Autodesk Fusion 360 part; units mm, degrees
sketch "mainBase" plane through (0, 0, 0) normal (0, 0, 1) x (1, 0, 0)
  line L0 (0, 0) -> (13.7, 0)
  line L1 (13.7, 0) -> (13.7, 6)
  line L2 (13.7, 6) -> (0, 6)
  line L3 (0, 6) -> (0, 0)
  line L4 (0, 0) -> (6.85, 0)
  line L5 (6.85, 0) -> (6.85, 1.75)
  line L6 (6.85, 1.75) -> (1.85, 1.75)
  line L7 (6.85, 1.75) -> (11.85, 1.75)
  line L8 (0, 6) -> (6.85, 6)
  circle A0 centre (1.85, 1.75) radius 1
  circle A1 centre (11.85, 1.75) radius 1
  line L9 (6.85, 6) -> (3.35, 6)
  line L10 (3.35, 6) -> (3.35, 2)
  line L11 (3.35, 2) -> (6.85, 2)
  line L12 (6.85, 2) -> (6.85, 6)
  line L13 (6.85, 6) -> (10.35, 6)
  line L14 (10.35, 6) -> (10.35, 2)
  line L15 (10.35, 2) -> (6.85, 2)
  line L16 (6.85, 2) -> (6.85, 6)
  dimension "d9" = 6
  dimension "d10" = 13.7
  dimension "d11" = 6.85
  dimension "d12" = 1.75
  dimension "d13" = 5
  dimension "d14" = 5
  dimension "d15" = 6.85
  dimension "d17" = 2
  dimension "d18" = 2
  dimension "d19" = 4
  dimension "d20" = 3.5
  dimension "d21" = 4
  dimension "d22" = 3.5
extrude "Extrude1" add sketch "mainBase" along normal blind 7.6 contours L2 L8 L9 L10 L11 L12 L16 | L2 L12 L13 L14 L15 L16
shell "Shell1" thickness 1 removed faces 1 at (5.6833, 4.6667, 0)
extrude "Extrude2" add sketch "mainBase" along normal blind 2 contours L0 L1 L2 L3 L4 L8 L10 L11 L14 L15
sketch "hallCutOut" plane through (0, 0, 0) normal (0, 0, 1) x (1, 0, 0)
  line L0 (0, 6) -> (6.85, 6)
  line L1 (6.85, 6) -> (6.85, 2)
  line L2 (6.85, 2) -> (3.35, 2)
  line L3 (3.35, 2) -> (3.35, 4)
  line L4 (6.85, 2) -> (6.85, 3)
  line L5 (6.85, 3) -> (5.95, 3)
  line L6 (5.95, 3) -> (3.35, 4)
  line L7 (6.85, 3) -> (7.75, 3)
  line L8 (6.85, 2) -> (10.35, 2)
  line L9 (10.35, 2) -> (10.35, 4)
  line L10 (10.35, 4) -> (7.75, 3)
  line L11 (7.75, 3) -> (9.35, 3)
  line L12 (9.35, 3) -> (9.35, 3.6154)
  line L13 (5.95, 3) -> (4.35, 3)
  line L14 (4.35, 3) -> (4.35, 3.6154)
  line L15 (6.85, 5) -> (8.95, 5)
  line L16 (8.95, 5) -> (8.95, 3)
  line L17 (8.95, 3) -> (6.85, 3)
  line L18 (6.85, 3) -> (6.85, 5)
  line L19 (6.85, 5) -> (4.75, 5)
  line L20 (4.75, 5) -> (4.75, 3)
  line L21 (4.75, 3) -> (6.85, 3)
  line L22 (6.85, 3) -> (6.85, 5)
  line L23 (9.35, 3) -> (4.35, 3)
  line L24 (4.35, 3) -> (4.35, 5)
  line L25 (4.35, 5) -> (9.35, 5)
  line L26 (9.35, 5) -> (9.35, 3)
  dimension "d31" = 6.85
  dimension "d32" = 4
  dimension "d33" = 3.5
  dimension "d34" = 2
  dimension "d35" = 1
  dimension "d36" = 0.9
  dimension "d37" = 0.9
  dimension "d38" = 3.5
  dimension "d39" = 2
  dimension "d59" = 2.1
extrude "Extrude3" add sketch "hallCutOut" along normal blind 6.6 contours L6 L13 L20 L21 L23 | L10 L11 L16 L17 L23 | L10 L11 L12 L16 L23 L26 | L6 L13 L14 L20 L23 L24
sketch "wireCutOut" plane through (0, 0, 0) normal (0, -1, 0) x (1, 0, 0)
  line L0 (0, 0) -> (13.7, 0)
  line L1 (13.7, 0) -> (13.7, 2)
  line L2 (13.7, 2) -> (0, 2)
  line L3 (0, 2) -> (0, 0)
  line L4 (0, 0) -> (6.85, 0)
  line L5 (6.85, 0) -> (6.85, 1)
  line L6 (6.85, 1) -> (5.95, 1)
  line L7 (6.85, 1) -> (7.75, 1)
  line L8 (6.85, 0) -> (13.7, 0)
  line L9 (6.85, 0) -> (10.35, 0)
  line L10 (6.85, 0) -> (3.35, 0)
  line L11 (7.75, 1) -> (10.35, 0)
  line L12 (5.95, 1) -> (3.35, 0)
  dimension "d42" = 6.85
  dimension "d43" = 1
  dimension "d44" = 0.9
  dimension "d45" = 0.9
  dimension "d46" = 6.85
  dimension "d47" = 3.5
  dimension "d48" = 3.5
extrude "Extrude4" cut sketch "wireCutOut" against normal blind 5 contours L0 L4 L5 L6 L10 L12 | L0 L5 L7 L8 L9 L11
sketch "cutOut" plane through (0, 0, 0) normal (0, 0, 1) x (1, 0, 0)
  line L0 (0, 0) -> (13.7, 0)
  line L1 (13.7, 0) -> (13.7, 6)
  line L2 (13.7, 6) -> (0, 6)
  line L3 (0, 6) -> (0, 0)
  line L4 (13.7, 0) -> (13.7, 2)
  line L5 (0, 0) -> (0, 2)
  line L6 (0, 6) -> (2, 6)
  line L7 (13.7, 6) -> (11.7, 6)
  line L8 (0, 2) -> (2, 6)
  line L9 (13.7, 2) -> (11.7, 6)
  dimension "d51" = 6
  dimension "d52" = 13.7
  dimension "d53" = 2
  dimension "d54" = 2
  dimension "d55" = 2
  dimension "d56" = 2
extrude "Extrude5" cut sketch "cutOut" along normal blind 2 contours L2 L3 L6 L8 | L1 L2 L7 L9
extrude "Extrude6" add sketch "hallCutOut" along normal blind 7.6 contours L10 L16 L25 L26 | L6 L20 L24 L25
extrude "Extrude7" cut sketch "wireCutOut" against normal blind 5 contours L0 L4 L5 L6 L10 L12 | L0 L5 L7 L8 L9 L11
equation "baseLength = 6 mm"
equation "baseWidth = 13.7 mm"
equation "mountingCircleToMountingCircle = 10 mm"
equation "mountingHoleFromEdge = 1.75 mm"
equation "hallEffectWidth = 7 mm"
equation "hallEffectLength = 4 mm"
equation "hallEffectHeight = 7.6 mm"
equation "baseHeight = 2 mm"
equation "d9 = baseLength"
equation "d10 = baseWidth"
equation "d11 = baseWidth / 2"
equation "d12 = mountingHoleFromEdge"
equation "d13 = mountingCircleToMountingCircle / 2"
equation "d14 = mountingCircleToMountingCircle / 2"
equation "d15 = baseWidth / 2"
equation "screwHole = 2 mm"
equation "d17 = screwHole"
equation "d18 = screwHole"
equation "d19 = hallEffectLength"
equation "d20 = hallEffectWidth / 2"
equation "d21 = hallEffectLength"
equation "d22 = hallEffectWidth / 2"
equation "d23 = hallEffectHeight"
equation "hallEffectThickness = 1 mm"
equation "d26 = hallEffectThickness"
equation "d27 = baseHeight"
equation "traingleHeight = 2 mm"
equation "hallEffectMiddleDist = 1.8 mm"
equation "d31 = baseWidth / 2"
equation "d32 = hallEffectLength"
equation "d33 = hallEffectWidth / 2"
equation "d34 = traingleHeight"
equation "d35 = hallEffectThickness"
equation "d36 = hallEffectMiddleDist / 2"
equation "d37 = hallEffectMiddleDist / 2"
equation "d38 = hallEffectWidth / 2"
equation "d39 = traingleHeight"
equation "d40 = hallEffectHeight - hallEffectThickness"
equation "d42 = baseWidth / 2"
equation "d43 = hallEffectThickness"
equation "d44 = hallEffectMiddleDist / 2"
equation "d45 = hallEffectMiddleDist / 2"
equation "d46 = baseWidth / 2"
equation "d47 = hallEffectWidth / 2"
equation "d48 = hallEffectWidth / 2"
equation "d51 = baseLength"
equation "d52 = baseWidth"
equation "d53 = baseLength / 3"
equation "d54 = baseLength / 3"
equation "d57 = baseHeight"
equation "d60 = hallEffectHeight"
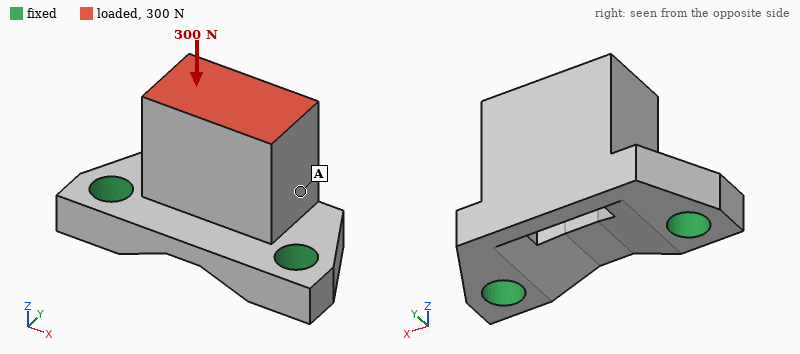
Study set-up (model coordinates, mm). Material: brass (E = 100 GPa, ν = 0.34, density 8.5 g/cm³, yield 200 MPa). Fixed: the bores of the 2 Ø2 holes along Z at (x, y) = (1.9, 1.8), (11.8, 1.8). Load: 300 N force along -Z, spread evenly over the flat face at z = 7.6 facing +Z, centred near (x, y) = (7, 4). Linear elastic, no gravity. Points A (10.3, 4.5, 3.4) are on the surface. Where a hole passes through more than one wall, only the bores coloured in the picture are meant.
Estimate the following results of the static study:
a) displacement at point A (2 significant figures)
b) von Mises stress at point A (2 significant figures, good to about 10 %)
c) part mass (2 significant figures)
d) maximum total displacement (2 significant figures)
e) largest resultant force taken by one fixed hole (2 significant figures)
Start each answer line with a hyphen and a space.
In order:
- 5.5 µm
- 26 MPa
- 1.9 g
- 11 µm
- 160 N
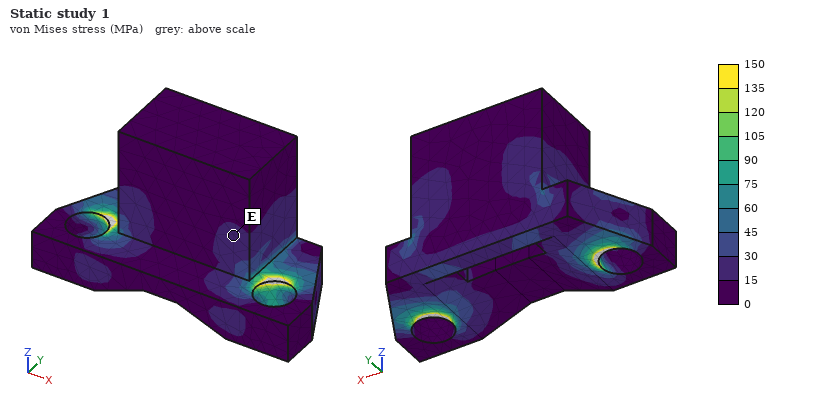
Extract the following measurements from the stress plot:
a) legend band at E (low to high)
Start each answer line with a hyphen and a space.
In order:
- 15 to 30 MPa
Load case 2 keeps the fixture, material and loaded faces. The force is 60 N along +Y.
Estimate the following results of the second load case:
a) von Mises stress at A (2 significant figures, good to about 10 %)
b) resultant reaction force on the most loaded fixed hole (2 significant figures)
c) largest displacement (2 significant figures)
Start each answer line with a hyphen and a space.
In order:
- 13 MPa
- 36 N
- 11 µm
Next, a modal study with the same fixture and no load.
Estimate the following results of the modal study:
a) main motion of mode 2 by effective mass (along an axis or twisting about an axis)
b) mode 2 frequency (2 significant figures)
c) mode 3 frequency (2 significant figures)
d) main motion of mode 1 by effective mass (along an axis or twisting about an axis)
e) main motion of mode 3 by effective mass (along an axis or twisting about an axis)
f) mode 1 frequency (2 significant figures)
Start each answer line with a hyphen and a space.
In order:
- along X
- 38 kHz
- 51 kHz
- along Y
- along Z
- 17 kHz
